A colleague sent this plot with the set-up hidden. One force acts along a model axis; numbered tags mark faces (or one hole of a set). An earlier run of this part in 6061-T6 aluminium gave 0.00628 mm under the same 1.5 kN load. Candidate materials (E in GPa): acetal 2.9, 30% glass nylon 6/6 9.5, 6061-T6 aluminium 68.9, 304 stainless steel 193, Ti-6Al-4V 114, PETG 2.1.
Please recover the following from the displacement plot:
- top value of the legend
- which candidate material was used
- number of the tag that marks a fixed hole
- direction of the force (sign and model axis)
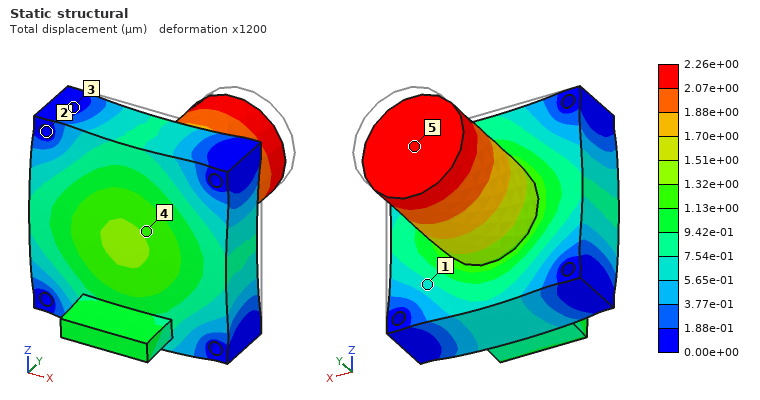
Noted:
2.26e+00 µm
304 stainless steel
2
-Y
